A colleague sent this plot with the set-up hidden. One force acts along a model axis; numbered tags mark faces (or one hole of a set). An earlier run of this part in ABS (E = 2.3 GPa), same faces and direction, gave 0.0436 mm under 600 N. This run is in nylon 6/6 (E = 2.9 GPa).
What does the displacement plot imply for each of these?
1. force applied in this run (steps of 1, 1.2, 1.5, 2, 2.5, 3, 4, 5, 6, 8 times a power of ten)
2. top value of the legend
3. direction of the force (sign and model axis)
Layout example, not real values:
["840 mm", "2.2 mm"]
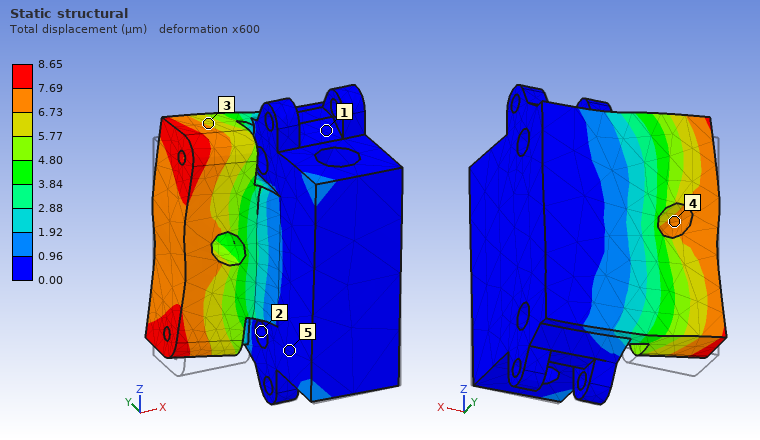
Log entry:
["150 N", "8.65 µm", "+Z"]
